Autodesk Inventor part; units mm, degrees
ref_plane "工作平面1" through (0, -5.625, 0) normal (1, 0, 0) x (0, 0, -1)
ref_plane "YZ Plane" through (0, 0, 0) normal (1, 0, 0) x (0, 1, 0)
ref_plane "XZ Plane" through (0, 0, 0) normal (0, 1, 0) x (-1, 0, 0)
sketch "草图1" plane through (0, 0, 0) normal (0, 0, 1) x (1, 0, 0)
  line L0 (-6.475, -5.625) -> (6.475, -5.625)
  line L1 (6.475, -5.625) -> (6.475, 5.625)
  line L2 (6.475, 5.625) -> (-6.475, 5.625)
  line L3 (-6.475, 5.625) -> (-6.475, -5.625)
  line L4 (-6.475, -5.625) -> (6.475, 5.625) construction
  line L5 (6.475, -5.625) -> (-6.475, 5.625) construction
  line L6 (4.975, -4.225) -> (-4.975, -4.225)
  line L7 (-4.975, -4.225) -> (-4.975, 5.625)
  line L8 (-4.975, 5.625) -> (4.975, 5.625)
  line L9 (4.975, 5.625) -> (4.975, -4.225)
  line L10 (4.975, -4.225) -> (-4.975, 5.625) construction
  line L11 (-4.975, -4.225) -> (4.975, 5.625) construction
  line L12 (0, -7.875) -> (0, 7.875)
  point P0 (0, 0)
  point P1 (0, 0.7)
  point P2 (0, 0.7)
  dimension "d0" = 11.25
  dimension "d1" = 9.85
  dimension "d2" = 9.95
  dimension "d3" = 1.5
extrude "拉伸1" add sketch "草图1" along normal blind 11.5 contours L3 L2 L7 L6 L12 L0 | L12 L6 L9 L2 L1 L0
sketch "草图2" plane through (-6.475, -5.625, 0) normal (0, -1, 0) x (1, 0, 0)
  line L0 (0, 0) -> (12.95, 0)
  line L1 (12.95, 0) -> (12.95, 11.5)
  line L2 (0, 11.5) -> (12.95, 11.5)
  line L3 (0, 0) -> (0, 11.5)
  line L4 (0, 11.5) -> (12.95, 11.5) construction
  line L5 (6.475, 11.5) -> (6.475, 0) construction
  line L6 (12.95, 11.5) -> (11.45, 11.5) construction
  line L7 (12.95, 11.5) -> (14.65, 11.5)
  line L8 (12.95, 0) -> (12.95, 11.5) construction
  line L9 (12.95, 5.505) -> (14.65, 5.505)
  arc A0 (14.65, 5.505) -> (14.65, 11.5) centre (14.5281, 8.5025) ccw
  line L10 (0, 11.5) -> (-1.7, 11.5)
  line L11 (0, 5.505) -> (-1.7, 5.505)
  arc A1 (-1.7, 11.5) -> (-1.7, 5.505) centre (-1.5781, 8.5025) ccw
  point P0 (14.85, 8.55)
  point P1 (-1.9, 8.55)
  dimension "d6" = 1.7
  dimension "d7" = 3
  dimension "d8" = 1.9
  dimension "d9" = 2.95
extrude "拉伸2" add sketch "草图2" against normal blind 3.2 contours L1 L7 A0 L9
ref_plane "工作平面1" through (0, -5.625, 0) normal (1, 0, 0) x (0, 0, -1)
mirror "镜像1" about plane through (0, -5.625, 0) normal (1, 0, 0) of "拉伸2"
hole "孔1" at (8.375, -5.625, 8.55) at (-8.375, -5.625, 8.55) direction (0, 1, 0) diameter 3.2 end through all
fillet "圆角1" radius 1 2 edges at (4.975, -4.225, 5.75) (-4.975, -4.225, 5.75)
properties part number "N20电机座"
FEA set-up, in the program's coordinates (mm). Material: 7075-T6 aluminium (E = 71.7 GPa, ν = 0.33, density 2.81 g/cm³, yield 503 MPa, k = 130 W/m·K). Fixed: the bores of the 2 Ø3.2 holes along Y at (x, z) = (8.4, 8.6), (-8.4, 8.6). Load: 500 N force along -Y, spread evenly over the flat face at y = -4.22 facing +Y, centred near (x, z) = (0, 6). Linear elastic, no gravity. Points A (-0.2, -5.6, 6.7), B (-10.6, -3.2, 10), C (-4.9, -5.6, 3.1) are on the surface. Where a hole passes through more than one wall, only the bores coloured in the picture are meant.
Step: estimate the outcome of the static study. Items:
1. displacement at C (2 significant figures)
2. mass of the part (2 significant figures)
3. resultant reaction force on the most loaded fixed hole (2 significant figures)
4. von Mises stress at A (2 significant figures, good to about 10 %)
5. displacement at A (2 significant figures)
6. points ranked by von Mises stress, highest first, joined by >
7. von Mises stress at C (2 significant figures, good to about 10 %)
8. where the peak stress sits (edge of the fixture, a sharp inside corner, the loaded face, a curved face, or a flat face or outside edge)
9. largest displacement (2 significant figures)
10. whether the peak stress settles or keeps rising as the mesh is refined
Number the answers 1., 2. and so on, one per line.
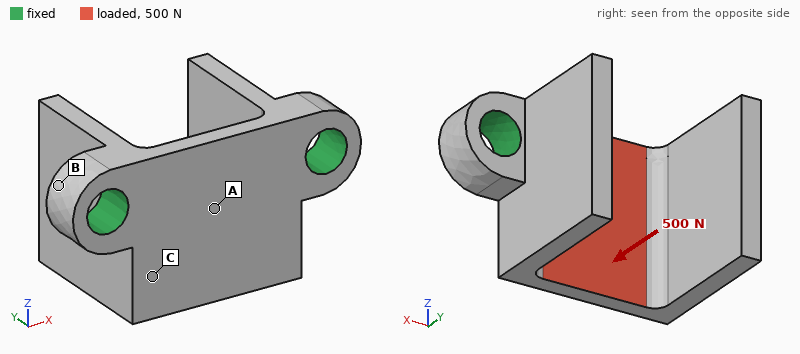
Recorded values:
1. 12 µm
2. 1.8 g
3. 280 N
4. 89 MPa
5. 19 µm
6. A > C > B
7. 40 MPa
8. edge of the fixture
9. 38 µm
10. keeps rising
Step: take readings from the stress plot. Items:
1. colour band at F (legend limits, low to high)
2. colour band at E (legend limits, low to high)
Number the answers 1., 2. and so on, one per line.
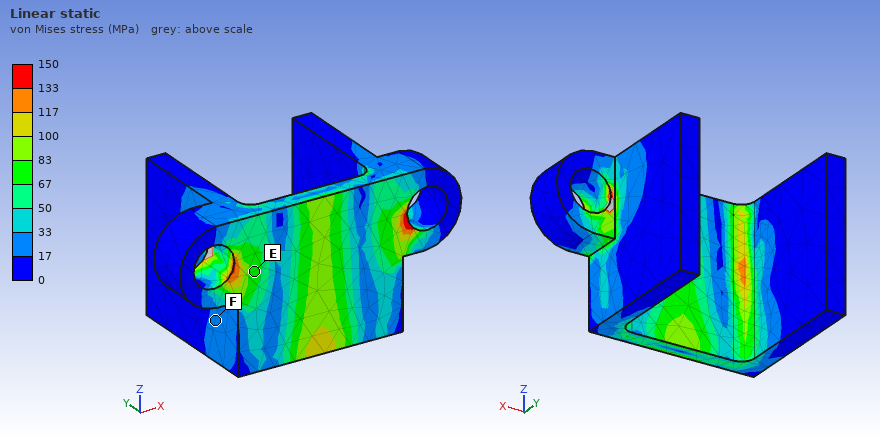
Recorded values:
1. 17 to 33 MPa
2. 67 to 83 MPa
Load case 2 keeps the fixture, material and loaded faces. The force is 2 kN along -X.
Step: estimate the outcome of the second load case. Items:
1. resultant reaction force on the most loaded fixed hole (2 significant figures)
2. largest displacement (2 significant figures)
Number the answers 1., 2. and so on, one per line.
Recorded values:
1. 1.1 kN
2. 18 µm
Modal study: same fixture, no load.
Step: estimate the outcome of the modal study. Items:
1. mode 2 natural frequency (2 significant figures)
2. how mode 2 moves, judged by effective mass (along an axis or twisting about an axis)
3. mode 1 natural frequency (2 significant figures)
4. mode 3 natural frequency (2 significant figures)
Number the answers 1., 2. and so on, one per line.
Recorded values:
1. 14 kHz
2. along X
3. 13 kHz
4. 22 kHz
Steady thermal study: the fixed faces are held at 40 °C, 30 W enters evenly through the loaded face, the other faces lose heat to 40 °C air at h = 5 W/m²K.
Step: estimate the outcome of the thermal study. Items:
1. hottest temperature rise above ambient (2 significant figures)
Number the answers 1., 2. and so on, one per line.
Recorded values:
1. 47 K
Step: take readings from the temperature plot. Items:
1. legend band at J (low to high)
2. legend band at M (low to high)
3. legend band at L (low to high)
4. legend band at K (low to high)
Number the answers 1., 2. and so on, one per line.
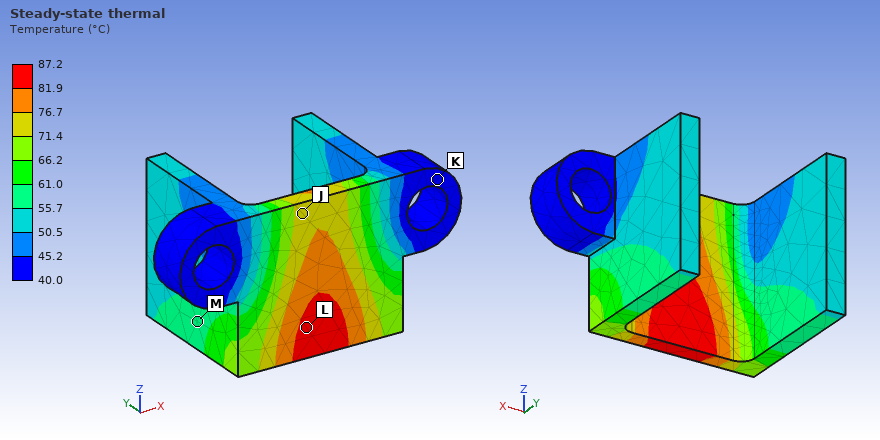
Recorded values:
1. 71.4 to 76.7 °C
2. 55.7 to 61.0 °C
3. 81.9 to 87.2 °C
4. 40.0 to 45.2 °C
